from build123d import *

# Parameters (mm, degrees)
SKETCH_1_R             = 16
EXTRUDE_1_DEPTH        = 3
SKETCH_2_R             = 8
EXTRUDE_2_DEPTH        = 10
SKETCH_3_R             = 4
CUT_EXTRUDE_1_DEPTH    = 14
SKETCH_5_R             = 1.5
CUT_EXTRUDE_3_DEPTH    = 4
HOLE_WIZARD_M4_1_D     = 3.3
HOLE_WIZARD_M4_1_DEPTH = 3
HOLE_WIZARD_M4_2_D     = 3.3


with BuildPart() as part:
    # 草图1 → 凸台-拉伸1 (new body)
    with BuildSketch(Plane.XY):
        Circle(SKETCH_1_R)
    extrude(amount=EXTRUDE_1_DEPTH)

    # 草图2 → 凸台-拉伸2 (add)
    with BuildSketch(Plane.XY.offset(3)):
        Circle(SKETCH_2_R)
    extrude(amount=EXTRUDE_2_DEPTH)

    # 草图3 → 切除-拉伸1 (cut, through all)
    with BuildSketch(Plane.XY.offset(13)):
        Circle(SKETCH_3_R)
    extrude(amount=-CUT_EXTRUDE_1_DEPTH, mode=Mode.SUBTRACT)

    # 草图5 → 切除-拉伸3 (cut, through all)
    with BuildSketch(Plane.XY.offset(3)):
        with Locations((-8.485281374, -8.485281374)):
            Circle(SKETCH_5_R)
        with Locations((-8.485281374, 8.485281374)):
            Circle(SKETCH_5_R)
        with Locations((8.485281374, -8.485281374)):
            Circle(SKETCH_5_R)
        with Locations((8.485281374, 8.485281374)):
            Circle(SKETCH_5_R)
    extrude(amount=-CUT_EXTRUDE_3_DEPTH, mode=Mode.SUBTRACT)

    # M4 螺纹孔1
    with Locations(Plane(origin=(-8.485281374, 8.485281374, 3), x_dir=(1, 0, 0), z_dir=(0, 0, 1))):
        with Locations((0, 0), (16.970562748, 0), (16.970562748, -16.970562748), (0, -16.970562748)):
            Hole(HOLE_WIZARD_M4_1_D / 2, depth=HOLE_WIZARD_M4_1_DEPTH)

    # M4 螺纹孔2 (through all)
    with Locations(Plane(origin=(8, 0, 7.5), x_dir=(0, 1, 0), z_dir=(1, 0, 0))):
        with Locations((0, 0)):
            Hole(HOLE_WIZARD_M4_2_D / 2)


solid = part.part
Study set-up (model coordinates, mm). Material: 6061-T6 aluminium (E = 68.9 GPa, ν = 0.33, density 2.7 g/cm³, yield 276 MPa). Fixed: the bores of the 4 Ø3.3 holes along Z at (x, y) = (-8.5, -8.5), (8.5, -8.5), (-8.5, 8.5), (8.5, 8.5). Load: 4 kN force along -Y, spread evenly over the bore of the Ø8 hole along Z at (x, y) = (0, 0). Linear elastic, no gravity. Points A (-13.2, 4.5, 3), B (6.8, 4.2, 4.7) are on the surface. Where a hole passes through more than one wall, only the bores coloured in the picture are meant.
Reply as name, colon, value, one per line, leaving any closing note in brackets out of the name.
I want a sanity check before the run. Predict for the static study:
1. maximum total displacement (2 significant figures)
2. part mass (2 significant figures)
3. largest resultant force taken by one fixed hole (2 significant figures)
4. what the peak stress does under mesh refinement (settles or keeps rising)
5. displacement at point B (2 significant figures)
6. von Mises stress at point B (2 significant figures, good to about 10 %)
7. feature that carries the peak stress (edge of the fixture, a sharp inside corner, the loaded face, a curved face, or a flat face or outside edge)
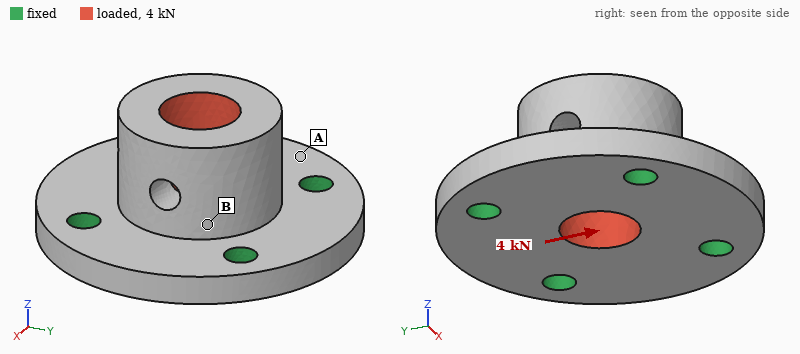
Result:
maximum total displacement: 30 µm
part mass: 9.7 g
largest resultant force taken by one fixed hole: 1.2 kN
what the peak stress does under mesh refinement: keeps rising
displacement at point B: 9.1 µm
von Mises stress at point B: 40 MPa
feature that carries the peak stress: edge of the fixture
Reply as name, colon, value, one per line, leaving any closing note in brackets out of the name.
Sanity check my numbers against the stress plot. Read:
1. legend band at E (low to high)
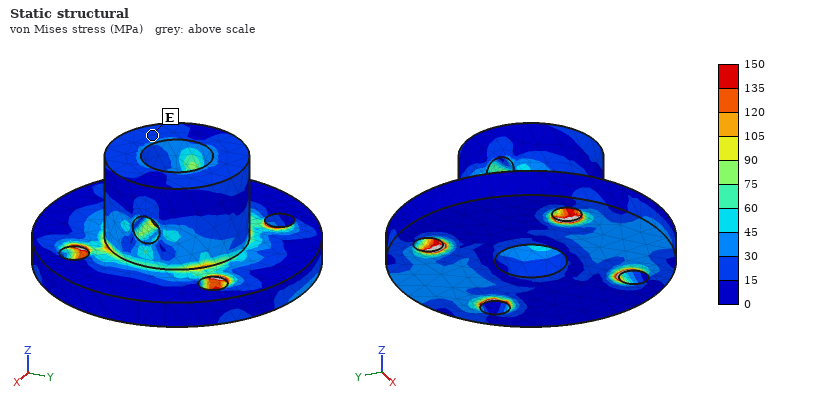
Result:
legend band at E: 15 to 30 MPa
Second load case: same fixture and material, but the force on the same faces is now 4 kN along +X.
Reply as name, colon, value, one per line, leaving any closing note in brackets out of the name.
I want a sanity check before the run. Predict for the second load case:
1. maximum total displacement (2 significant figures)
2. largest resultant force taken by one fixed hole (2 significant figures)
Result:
maximum total displacement: 28 µm
largest resultant force taken by one fixed hole: 1.2 kN
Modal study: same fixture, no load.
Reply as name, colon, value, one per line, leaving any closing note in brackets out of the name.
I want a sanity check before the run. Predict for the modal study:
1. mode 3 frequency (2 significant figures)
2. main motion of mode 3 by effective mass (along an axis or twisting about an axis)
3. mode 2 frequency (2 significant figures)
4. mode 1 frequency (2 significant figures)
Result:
mode 3 frequency: 35 kHz
main motion of mode 3 by effective mass: along Z
mode 2 frequency: 30 kHz
mode 1 frequency: 29 kHz
